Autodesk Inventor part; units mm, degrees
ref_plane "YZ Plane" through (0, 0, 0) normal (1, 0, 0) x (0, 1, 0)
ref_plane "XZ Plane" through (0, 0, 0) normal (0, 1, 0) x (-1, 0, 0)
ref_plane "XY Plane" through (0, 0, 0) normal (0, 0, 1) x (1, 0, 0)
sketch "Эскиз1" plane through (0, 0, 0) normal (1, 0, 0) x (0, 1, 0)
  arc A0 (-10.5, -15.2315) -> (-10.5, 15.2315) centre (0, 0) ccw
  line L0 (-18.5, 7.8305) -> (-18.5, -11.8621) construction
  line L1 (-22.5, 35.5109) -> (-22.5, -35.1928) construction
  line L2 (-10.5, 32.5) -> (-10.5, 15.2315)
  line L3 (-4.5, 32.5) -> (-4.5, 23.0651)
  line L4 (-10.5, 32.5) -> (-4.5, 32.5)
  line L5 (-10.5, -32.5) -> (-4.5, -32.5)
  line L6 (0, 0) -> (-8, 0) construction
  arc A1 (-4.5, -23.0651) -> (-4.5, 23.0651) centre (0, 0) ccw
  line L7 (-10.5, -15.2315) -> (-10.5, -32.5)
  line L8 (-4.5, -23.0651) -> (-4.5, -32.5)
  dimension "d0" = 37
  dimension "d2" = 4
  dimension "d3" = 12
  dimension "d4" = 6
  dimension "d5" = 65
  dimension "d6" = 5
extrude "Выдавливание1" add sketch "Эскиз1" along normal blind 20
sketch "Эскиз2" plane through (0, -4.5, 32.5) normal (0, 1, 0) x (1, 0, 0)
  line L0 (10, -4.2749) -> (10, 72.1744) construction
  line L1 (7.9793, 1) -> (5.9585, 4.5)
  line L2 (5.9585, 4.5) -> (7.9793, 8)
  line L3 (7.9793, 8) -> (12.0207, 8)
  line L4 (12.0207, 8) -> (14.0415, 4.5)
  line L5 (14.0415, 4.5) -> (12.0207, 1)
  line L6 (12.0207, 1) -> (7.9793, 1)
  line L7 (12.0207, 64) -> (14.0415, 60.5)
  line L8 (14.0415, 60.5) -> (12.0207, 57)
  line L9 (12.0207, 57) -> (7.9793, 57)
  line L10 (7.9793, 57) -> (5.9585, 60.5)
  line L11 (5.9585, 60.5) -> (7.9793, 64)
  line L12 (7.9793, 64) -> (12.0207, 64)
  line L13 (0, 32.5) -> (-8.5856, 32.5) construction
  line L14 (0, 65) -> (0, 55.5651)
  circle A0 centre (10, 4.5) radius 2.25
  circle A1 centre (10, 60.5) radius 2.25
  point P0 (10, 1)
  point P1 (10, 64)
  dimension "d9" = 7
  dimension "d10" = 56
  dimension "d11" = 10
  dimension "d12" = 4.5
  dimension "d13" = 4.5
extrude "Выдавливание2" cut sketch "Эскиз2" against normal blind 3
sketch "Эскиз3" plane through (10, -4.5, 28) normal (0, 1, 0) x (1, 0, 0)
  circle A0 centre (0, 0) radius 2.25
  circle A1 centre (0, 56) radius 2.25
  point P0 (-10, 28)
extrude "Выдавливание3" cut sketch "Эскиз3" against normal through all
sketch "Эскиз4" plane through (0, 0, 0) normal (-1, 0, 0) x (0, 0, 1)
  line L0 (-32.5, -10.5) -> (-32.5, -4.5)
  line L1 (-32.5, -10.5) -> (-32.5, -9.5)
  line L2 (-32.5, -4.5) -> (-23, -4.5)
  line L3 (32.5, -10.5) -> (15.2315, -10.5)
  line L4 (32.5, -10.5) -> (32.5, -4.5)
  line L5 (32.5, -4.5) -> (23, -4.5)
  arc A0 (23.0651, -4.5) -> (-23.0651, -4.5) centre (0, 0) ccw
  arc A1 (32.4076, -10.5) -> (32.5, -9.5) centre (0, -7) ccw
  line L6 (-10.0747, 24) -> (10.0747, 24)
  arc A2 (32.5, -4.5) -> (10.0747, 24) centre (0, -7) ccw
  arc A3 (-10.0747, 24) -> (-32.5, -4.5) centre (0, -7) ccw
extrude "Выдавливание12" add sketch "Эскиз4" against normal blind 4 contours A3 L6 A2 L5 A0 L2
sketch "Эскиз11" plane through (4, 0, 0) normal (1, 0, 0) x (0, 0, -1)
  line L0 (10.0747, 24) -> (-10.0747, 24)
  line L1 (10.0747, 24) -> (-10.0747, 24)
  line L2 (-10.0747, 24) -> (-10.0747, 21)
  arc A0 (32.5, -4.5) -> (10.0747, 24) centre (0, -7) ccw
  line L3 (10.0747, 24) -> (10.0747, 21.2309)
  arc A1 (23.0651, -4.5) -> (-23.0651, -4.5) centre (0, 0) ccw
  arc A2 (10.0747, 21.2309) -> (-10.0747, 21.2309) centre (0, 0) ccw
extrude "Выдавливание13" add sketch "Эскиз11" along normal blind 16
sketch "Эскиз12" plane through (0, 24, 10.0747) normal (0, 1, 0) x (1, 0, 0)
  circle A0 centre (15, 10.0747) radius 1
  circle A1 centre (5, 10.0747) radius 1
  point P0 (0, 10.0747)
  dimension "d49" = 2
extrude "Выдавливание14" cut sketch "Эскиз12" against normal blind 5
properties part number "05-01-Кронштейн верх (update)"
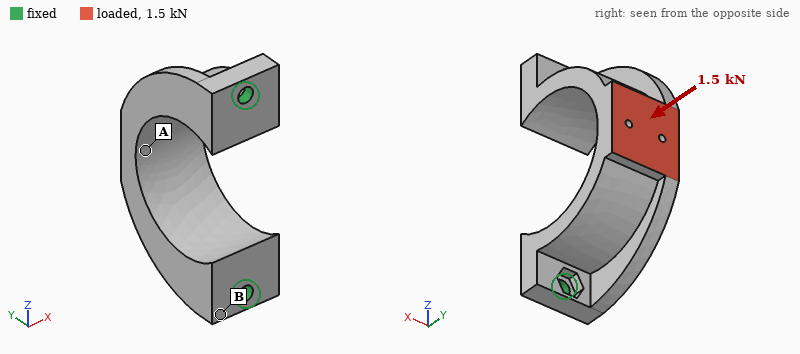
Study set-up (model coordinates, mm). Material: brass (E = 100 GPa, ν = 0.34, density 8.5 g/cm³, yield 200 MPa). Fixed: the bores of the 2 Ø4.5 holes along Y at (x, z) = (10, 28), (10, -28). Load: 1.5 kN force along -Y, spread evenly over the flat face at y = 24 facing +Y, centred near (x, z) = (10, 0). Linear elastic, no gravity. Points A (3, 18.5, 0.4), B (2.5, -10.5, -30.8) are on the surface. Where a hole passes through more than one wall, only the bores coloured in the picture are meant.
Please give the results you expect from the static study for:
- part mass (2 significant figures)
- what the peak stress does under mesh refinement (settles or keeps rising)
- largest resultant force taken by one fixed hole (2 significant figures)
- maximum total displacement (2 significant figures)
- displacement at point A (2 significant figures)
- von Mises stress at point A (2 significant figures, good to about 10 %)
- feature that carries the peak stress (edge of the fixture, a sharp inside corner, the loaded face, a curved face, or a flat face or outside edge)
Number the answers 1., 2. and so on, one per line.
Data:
1. 110 g
2. keeps rising
3. 870 N
4. 16 µm
5. 12 µm
6. 25 MPa
7. edge of the fixture
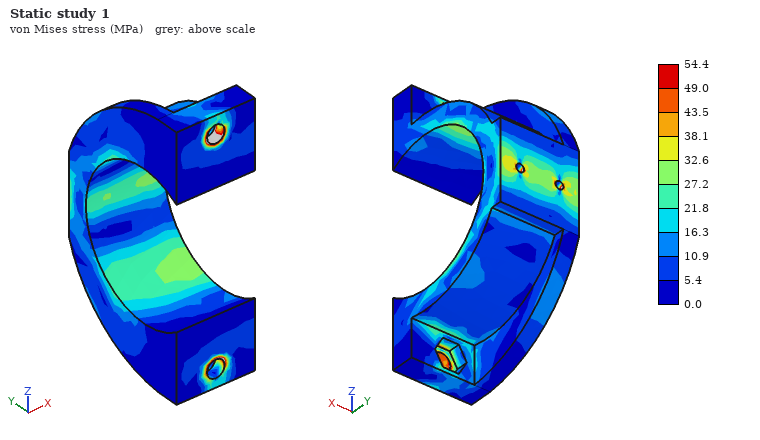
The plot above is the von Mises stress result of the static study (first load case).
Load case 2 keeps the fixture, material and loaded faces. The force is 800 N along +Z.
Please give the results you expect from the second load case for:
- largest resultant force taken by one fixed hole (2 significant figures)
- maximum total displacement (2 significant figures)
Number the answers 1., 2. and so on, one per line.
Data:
1. 580 N
2. 24 µm
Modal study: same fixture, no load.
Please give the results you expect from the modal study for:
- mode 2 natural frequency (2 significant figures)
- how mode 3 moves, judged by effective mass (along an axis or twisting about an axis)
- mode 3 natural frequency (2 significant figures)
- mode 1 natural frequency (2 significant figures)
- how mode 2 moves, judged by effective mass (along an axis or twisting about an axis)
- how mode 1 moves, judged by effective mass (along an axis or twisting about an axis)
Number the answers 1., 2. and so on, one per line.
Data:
1. 3700 Hz
2. twisting about Y
3. 5100 Hz
4. 1800 Hz
5. along Z
6. along X
